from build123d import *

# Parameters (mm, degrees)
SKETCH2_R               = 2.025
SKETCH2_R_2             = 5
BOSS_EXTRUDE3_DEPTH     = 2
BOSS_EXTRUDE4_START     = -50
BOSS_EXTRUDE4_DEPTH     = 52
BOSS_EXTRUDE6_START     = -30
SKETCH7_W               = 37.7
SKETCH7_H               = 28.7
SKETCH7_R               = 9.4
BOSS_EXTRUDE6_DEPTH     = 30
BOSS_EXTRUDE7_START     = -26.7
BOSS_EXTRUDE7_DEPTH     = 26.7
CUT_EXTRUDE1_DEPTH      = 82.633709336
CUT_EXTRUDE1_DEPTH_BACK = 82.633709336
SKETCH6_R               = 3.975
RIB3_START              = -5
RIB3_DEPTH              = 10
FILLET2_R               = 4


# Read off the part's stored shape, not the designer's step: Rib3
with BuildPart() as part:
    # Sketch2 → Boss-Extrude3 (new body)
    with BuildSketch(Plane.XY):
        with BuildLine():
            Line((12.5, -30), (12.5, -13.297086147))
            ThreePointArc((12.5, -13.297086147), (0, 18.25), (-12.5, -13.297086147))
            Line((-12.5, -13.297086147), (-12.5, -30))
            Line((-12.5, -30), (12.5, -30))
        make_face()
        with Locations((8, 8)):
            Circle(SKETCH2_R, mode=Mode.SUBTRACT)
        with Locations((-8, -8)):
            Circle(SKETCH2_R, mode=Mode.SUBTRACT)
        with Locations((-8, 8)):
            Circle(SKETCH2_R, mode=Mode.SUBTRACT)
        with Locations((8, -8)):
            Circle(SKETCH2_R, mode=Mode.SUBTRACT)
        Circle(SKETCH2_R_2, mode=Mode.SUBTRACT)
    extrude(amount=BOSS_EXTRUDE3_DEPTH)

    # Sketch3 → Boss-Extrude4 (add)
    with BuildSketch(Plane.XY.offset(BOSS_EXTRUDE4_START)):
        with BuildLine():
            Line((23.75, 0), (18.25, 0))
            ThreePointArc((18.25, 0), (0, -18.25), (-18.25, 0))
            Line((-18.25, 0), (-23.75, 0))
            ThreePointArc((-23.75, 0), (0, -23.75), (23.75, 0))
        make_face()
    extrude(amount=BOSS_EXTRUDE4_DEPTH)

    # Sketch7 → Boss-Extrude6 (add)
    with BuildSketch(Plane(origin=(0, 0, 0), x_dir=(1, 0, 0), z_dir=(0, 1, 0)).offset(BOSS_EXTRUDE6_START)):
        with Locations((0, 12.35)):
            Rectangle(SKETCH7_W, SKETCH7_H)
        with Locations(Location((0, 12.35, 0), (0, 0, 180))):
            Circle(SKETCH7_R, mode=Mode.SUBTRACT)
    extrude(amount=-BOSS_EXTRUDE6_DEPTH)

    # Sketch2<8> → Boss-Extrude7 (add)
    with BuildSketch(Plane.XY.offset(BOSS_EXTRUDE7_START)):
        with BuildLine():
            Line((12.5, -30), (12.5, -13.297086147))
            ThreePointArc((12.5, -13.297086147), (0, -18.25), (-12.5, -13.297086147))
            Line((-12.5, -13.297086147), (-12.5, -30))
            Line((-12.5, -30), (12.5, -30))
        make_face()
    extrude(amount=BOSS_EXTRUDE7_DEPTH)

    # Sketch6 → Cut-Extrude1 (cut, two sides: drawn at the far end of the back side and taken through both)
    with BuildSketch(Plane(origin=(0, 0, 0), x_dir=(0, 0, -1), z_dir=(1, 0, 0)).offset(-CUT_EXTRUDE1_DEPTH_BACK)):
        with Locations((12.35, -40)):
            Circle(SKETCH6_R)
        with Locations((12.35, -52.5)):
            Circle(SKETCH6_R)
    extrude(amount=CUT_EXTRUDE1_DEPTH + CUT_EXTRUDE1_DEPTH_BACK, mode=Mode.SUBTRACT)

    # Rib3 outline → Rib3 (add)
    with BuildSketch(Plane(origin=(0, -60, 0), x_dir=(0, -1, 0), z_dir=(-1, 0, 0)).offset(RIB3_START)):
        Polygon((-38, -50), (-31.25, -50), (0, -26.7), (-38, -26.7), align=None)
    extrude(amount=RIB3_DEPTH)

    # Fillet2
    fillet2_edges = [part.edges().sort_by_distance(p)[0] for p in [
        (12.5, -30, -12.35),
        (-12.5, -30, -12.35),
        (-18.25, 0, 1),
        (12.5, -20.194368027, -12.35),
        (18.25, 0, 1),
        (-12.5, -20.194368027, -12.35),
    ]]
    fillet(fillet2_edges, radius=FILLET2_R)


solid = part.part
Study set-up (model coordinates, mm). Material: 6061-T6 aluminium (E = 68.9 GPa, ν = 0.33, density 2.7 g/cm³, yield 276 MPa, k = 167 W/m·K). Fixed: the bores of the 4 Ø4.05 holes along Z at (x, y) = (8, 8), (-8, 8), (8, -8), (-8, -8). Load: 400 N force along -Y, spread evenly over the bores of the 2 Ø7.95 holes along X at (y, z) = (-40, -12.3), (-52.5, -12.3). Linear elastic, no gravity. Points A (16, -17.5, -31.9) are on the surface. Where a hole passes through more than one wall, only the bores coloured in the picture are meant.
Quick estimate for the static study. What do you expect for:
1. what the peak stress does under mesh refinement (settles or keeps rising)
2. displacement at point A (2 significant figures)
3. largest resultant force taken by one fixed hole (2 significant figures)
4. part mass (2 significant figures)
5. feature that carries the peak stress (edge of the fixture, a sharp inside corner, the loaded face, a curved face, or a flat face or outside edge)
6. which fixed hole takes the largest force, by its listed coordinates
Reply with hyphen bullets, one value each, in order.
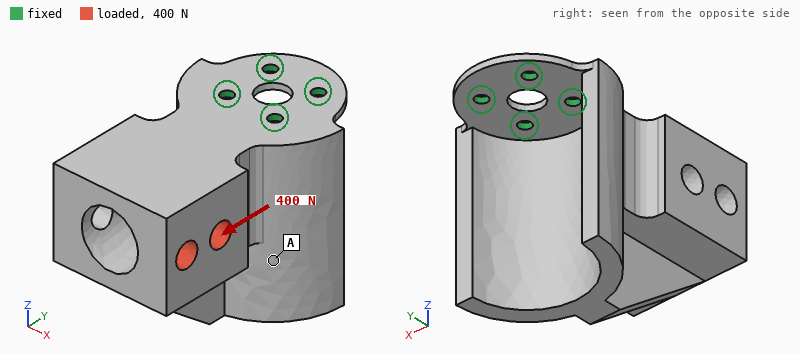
- keeps rising
- 0.16 mm
- 340 N
- 140 g
- edge of the fixture
- (8, -8)
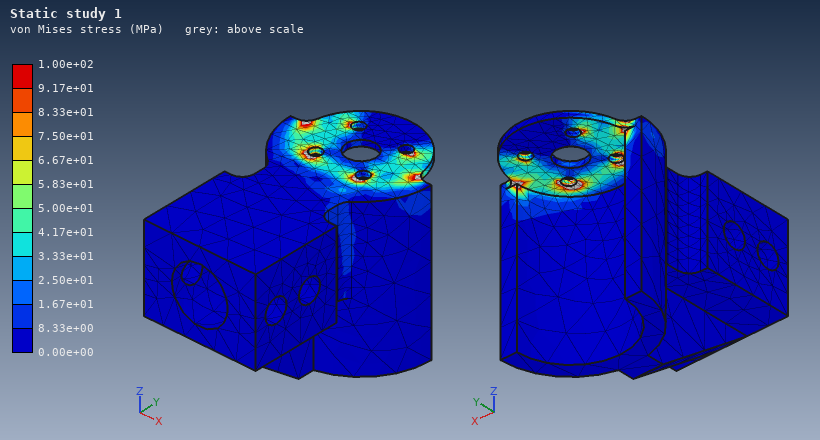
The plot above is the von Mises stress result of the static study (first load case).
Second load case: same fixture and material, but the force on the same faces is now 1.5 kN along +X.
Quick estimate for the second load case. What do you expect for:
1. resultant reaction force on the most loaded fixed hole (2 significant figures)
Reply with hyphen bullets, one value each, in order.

- 2.3 kN
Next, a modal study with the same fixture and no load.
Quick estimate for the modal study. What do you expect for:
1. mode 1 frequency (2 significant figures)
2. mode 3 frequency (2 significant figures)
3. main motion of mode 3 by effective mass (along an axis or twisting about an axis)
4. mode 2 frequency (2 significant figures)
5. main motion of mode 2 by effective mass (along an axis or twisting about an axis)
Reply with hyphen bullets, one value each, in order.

- 400 Hz
- 2800 Hz
- along X
- 1200 Hz
- along X
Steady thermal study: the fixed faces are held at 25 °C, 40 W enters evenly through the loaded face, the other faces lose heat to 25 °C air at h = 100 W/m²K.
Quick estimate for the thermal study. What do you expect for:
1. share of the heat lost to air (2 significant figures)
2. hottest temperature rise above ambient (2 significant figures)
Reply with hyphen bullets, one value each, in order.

- 57 %
- 24 K
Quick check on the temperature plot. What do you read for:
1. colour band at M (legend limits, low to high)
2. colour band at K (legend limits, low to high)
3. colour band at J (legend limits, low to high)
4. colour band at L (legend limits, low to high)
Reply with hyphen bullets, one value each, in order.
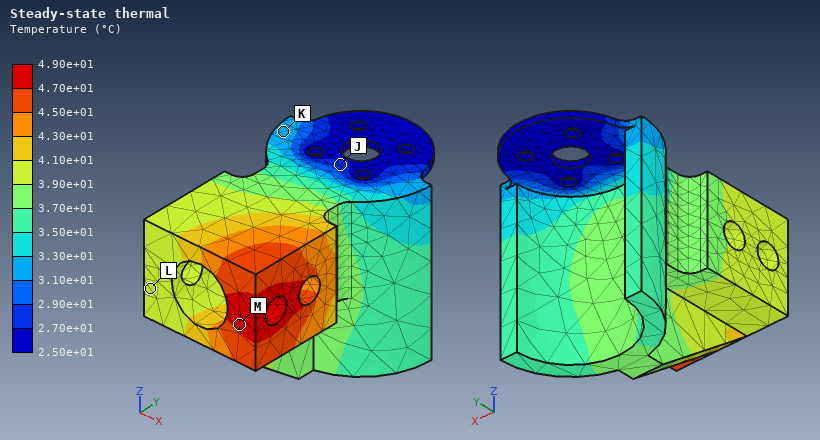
- 4.70e+01 to 4.90e+01 °C
- 3.10e+01 to 3.30e+01 °C
- 2.70e+01 to 2.90e+01 °C
- 3.90e+01 to 4.10e+01 °C
